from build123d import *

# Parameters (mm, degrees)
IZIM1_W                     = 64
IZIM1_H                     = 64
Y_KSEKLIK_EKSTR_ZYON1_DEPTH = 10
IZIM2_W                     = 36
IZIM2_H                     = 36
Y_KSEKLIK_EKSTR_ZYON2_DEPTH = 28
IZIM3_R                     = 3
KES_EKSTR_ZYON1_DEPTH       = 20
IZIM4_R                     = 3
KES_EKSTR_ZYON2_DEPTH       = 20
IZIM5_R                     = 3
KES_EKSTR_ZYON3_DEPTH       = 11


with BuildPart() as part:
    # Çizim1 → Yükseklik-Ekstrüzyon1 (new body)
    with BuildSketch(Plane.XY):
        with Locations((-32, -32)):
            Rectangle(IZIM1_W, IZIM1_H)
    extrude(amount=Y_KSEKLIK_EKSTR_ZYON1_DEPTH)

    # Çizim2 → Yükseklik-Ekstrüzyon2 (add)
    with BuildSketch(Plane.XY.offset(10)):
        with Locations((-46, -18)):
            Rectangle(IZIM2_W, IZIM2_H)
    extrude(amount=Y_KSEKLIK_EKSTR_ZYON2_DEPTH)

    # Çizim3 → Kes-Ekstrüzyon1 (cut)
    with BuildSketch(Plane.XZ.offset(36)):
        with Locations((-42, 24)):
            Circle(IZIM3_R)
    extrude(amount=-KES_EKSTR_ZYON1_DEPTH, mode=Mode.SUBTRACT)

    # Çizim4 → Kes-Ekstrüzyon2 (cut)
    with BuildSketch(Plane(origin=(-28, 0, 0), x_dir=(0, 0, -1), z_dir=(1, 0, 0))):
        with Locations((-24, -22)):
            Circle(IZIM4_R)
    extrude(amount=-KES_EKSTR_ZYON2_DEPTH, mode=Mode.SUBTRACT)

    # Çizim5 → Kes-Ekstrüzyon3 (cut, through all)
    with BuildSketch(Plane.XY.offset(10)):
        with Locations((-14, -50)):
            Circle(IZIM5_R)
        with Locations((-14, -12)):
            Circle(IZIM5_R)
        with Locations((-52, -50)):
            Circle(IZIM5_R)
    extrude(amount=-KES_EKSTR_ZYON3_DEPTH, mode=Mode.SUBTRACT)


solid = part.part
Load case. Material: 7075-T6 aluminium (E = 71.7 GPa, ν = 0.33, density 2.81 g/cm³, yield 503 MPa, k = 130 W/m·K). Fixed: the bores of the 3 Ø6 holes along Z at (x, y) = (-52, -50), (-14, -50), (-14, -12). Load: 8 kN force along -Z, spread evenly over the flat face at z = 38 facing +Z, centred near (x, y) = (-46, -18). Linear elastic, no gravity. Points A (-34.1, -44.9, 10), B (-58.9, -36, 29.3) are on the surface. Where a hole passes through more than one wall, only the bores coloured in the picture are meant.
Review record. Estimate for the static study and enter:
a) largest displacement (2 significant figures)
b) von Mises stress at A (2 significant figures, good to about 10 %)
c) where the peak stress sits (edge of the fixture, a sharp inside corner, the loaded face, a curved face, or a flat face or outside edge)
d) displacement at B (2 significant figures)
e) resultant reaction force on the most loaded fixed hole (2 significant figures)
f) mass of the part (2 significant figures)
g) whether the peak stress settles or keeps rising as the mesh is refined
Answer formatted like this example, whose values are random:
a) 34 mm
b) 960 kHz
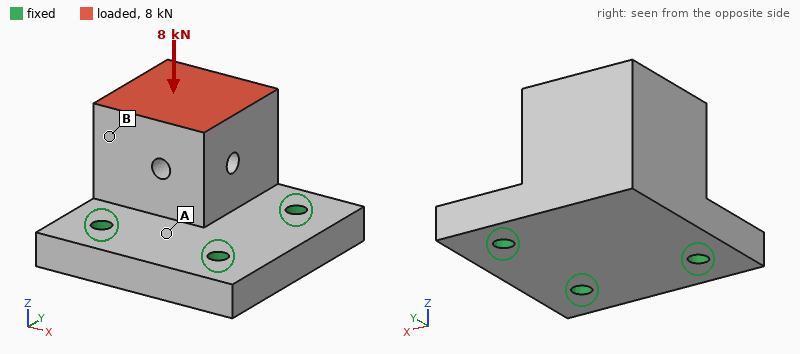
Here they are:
a) 0.19 mm
b) 38 MPa
c) edge of the fixture
d) 0.097 mm
e) 4.9 kN
f) 210 g
g) keeps rising
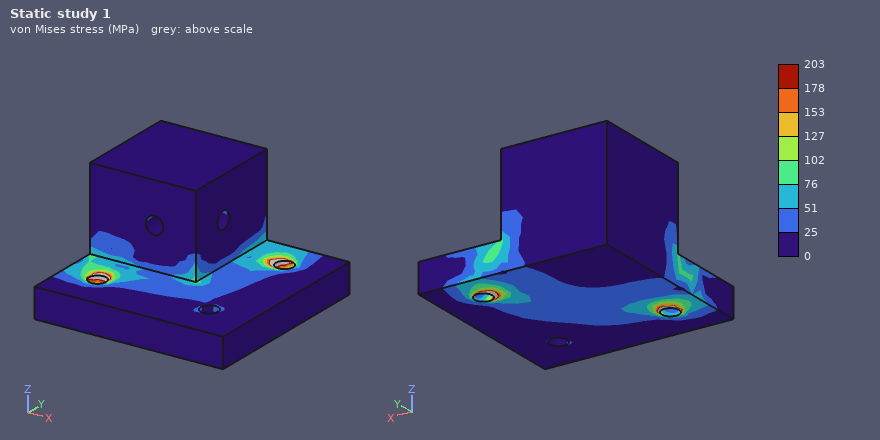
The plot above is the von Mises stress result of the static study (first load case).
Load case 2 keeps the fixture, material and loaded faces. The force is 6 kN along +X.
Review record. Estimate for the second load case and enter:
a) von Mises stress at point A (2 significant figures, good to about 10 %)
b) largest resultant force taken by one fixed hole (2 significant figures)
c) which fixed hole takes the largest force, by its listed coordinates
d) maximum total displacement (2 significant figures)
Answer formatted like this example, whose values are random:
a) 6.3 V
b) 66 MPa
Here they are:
a) 48 MPa
b) 4.8 kN
c) (-52, -50)
d) 0.20 mm
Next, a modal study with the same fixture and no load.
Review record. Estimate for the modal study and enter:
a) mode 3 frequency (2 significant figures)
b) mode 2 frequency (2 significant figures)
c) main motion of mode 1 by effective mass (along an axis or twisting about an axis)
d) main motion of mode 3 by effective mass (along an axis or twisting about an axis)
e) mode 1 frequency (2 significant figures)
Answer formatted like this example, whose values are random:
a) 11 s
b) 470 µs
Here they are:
a) 10000 Hz
b) 7400 Hz
c) along Z
d) along Z
e) 3200 Hz
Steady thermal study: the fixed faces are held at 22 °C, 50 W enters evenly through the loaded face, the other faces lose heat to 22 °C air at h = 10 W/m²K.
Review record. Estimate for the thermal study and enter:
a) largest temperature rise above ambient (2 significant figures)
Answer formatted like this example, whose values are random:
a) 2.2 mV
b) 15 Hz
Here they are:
a) 22 K
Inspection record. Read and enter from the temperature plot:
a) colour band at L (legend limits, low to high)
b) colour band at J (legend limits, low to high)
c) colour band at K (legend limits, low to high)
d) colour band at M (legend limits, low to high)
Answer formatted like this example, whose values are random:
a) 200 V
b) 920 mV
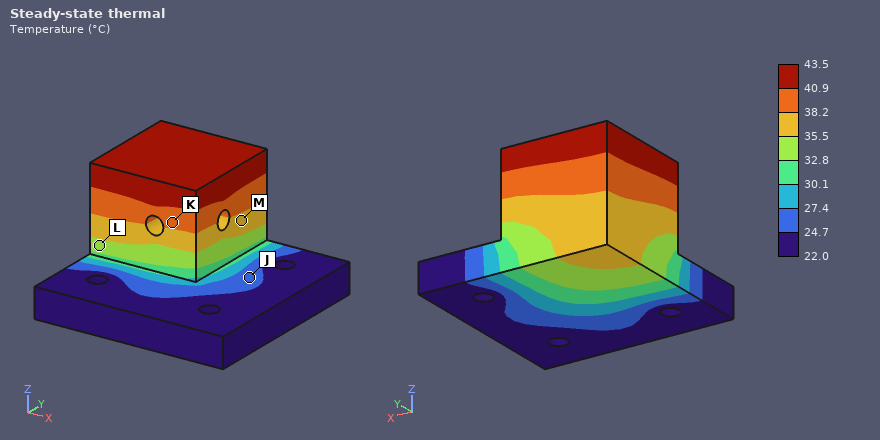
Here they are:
a) 32.8 to 35.5 °C
b) 24.7 to 27.4 °C
c) 38.2 to 40.9 °C
d) 35.5 to 38.2 °C
